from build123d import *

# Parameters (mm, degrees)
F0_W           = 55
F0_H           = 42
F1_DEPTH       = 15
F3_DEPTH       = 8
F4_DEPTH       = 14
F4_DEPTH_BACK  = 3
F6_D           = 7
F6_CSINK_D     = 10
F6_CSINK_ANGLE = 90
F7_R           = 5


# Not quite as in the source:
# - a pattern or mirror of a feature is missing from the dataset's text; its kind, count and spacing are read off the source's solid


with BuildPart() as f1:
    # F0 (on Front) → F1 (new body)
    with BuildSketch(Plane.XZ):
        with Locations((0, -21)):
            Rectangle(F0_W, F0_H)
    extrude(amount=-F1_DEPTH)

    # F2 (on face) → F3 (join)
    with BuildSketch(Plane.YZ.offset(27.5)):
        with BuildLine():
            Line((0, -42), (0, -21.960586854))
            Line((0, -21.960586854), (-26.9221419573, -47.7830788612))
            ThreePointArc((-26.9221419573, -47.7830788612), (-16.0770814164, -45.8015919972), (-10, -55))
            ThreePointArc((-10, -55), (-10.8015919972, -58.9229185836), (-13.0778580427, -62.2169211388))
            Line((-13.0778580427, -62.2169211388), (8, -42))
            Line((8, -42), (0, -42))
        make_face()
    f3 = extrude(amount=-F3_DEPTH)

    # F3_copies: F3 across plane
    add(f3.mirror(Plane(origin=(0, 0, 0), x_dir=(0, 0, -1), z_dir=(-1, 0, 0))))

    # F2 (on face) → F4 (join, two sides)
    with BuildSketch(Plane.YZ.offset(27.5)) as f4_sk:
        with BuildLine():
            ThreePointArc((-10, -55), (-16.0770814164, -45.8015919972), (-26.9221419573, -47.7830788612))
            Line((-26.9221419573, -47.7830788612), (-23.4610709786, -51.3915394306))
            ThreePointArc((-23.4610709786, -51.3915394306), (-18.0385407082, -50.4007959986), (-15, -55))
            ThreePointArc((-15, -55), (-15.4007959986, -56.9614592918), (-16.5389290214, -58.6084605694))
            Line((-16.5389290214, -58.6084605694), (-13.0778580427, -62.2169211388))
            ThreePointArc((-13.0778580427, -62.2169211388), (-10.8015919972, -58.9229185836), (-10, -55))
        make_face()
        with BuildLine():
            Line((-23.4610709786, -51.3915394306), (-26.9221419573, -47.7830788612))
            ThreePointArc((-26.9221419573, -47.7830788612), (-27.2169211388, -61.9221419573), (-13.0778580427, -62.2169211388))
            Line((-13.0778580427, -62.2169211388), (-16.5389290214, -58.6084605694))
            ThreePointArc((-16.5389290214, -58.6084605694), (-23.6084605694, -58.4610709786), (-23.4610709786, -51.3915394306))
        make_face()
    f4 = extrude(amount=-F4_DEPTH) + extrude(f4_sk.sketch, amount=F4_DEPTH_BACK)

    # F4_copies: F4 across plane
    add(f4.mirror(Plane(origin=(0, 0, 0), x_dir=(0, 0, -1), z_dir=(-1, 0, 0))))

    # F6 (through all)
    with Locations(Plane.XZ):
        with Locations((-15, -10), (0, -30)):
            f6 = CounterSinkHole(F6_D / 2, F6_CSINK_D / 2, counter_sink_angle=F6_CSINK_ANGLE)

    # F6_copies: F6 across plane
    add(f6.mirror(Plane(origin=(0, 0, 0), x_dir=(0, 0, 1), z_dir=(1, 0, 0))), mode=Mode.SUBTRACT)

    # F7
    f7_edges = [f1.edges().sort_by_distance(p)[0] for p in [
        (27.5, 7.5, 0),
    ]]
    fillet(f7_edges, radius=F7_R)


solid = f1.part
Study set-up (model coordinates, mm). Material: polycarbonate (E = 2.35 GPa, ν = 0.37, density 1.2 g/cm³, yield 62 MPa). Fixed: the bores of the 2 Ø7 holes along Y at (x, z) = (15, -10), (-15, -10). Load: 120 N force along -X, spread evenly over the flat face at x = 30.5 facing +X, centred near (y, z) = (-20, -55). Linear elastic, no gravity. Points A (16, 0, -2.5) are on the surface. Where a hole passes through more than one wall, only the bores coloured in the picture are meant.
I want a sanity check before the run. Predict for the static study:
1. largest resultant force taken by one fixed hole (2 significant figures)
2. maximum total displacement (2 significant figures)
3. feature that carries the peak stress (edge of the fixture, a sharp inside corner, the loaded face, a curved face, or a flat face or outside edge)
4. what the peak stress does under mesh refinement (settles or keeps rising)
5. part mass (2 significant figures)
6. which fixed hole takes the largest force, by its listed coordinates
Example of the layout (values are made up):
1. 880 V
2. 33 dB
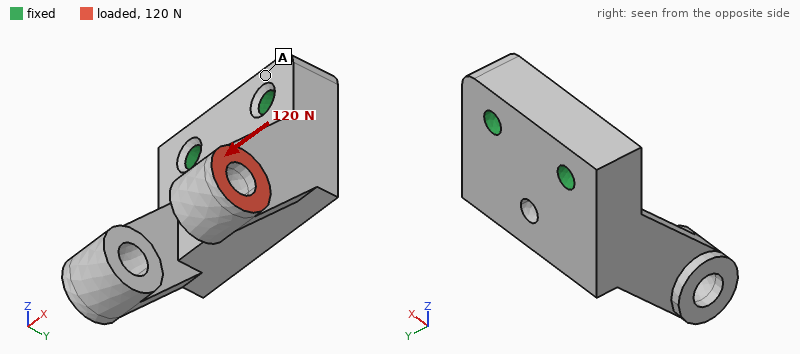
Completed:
1. 190 N
2. 1.0 mm
3. a sharp inside corner
4. keeps rising
5. 57 g
6. (-15, -10)
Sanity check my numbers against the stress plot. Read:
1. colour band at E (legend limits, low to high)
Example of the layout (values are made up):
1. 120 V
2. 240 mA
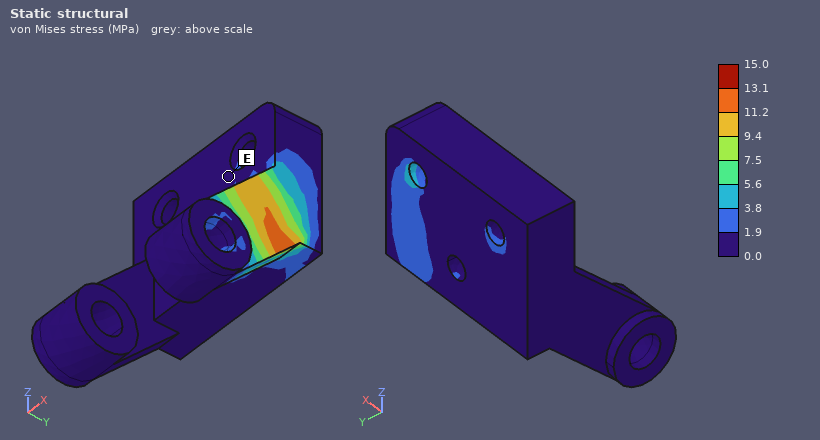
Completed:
1. 0.0 to 1.9 MPa
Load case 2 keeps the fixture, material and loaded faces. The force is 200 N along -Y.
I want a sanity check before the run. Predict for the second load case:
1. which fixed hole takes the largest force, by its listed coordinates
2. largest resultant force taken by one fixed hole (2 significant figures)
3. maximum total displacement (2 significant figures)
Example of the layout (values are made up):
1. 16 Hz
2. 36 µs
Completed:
1. (15, -10)
2. 240 N
3. 1.0 mm
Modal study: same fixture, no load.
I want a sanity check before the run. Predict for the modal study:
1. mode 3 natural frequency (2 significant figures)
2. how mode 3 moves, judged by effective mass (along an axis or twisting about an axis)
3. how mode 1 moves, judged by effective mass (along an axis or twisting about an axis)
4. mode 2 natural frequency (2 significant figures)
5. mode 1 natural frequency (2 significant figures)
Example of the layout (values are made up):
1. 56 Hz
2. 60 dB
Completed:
1. 970 Hz
2. along Y
3. along X
4. 870 Hz
5. 830 Hz
